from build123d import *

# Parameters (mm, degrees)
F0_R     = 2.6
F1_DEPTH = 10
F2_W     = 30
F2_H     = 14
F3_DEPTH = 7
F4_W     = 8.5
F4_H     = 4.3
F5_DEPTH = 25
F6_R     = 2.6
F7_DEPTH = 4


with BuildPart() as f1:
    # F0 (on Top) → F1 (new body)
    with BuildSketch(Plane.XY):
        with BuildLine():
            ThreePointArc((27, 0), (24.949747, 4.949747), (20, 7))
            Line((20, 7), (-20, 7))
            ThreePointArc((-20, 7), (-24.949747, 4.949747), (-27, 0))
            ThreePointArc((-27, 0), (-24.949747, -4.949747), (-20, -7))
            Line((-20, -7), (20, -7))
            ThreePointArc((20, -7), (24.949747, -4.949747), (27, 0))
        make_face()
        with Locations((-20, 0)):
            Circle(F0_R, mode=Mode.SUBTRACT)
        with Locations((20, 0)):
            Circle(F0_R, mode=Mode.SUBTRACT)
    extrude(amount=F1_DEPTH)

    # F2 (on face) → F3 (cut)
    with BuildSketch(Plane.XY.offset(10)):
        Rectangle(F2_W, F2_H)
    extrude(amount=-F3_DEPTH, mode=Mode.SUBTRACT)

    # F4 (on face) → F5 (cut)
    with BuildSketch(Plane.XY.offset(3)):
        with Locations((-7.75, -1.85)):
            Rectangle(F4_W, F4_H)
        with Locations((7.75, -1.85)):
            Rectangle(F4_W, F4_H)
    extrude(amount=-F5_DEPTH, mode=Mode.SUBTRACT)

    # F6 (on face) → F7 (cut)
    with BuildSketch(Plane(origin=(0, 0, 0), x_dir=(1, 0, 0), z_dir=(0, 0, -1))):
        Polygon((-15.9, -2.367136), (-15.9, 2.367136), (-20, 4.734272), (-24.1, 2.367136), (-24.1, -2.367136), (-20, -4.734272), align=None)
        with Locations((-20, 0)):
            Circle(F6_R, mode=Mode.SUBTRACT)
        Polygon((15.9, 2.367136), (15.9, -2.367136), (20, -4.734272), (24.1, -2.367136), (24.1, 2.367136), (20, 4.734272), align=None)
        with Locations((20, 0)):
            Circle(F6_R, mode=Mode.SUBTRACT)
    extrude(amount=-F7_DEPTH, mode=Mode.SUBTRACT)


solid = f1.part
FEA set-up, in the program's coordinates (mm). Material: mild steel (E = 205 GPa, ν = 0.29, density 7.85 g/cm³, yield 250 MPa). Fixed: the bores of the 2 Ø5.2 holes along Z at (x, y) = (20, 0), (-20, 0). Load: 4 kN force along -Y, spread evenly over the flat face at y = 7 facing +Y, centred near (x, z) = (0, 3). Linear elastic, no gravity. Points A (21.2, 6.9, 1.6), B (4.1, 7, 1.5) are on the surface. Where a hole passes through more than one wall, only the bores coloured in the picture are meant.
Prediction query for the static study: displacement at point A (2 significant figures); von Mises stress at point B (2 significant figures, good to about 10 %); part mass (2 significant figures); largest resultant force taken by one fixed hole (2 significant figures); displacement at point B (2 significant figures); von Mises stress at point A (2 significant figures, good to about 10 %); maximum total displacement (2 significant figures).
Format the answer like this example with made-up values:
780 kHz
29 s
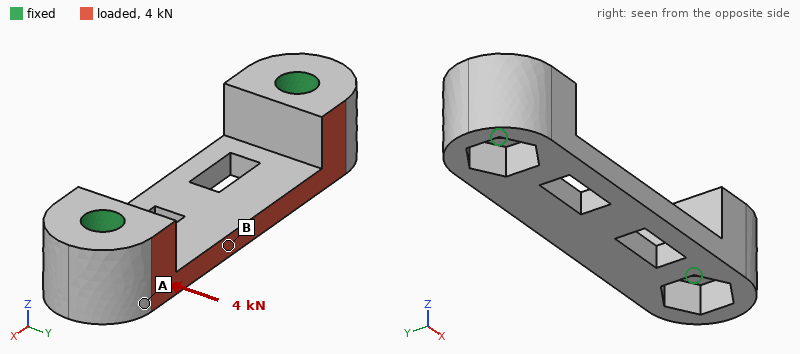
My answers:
3.0 µm
92 MPa
26 g
2.0 kN
17 µm
25 MPa
18 µm
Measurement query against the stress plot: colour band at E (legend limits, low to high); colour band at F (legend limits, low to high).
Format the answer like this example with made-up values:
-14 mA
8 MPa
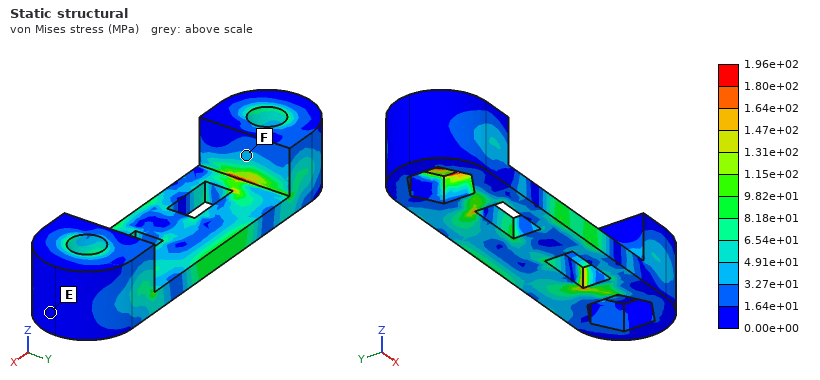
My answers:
0.00e+00 to 1.64e+01 MPa
3.27e+01 to 4.91e+01 MPa
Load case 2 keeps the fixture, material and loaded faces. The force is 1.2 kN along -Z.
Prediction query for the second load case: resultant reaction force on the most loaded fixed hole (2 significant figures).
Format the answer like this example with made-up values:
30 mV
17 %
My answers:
650 N
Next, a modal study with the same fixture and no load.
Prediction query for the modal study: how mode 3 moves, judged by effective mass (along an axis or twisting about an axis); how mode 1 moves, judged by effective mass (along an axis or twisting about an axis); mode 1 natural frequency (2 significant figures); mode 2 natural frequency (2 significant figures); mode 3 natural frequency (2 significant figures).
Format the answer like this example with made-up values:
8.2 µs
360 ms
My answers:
along Y
along Z
13 kHz
19 kHz
21 kHz
